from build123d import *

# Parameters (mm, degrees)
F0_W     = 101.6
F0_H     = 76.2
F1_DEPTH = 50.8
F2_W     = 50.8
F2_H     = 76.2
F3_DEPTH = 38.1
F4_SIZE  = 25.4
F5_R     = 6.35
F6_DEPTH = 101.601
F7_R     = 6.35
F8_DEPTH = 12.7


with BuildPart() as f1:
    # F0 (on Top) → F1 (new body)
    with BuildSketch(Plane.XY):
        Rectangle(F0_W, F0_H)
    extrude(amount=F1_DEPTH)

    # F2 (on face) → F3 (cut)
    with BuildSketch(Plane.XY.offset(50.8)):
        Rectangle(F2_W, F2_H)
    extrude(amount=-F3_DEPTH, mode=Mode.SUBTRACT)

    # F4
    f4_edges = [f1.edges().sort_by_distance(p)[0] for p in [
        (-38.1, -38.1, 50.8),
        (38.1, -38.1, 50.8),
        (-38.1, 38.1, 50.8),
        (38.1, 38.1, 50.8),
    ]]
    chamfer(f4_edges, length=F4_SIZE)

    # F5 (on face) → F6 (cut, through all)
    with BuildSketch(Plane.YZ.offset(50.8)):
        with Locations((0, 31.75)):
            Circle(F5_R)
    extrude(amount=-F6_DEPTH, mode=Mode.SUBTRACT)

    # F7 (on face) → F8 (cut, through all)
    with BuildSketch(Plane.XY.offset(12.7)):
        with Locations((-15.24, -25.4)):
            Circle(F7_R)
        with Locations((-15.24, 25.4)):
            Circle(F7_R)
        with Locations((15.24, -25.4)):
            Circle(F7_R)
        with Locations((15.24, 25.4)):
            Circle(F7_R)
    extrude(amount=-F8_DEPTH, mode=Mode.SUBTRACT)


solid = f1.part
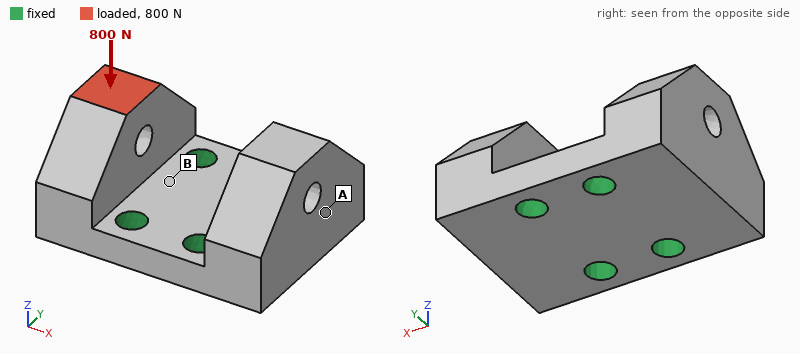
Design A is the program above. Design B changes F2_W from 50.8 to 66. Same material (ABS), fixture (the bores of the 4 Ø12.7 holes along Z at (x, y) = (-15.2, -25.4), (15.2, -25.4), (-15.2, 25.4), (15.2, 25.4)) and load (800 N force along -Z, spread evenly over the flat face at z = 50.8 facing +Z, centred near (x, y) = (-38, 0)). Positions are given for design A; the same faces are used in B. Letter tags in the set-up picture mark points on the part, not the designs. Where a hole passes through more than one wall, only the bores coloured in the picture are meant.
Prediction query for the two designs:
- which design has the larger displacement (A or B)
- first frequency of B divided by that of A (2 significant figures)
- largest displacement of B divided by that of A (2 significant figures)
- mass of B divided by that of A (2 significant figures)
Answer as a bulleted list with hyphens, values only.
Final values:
- B
- 0.97
- 1.5
- 0.84
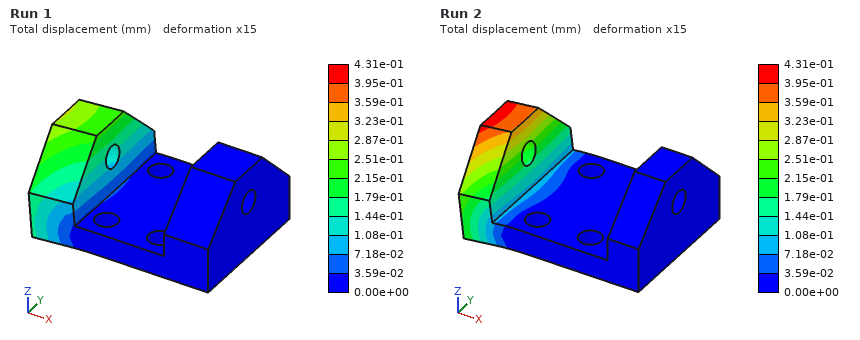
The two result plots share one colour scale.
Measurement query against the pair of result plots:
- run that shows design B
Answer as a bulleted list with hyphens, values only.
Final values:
- Run 2
